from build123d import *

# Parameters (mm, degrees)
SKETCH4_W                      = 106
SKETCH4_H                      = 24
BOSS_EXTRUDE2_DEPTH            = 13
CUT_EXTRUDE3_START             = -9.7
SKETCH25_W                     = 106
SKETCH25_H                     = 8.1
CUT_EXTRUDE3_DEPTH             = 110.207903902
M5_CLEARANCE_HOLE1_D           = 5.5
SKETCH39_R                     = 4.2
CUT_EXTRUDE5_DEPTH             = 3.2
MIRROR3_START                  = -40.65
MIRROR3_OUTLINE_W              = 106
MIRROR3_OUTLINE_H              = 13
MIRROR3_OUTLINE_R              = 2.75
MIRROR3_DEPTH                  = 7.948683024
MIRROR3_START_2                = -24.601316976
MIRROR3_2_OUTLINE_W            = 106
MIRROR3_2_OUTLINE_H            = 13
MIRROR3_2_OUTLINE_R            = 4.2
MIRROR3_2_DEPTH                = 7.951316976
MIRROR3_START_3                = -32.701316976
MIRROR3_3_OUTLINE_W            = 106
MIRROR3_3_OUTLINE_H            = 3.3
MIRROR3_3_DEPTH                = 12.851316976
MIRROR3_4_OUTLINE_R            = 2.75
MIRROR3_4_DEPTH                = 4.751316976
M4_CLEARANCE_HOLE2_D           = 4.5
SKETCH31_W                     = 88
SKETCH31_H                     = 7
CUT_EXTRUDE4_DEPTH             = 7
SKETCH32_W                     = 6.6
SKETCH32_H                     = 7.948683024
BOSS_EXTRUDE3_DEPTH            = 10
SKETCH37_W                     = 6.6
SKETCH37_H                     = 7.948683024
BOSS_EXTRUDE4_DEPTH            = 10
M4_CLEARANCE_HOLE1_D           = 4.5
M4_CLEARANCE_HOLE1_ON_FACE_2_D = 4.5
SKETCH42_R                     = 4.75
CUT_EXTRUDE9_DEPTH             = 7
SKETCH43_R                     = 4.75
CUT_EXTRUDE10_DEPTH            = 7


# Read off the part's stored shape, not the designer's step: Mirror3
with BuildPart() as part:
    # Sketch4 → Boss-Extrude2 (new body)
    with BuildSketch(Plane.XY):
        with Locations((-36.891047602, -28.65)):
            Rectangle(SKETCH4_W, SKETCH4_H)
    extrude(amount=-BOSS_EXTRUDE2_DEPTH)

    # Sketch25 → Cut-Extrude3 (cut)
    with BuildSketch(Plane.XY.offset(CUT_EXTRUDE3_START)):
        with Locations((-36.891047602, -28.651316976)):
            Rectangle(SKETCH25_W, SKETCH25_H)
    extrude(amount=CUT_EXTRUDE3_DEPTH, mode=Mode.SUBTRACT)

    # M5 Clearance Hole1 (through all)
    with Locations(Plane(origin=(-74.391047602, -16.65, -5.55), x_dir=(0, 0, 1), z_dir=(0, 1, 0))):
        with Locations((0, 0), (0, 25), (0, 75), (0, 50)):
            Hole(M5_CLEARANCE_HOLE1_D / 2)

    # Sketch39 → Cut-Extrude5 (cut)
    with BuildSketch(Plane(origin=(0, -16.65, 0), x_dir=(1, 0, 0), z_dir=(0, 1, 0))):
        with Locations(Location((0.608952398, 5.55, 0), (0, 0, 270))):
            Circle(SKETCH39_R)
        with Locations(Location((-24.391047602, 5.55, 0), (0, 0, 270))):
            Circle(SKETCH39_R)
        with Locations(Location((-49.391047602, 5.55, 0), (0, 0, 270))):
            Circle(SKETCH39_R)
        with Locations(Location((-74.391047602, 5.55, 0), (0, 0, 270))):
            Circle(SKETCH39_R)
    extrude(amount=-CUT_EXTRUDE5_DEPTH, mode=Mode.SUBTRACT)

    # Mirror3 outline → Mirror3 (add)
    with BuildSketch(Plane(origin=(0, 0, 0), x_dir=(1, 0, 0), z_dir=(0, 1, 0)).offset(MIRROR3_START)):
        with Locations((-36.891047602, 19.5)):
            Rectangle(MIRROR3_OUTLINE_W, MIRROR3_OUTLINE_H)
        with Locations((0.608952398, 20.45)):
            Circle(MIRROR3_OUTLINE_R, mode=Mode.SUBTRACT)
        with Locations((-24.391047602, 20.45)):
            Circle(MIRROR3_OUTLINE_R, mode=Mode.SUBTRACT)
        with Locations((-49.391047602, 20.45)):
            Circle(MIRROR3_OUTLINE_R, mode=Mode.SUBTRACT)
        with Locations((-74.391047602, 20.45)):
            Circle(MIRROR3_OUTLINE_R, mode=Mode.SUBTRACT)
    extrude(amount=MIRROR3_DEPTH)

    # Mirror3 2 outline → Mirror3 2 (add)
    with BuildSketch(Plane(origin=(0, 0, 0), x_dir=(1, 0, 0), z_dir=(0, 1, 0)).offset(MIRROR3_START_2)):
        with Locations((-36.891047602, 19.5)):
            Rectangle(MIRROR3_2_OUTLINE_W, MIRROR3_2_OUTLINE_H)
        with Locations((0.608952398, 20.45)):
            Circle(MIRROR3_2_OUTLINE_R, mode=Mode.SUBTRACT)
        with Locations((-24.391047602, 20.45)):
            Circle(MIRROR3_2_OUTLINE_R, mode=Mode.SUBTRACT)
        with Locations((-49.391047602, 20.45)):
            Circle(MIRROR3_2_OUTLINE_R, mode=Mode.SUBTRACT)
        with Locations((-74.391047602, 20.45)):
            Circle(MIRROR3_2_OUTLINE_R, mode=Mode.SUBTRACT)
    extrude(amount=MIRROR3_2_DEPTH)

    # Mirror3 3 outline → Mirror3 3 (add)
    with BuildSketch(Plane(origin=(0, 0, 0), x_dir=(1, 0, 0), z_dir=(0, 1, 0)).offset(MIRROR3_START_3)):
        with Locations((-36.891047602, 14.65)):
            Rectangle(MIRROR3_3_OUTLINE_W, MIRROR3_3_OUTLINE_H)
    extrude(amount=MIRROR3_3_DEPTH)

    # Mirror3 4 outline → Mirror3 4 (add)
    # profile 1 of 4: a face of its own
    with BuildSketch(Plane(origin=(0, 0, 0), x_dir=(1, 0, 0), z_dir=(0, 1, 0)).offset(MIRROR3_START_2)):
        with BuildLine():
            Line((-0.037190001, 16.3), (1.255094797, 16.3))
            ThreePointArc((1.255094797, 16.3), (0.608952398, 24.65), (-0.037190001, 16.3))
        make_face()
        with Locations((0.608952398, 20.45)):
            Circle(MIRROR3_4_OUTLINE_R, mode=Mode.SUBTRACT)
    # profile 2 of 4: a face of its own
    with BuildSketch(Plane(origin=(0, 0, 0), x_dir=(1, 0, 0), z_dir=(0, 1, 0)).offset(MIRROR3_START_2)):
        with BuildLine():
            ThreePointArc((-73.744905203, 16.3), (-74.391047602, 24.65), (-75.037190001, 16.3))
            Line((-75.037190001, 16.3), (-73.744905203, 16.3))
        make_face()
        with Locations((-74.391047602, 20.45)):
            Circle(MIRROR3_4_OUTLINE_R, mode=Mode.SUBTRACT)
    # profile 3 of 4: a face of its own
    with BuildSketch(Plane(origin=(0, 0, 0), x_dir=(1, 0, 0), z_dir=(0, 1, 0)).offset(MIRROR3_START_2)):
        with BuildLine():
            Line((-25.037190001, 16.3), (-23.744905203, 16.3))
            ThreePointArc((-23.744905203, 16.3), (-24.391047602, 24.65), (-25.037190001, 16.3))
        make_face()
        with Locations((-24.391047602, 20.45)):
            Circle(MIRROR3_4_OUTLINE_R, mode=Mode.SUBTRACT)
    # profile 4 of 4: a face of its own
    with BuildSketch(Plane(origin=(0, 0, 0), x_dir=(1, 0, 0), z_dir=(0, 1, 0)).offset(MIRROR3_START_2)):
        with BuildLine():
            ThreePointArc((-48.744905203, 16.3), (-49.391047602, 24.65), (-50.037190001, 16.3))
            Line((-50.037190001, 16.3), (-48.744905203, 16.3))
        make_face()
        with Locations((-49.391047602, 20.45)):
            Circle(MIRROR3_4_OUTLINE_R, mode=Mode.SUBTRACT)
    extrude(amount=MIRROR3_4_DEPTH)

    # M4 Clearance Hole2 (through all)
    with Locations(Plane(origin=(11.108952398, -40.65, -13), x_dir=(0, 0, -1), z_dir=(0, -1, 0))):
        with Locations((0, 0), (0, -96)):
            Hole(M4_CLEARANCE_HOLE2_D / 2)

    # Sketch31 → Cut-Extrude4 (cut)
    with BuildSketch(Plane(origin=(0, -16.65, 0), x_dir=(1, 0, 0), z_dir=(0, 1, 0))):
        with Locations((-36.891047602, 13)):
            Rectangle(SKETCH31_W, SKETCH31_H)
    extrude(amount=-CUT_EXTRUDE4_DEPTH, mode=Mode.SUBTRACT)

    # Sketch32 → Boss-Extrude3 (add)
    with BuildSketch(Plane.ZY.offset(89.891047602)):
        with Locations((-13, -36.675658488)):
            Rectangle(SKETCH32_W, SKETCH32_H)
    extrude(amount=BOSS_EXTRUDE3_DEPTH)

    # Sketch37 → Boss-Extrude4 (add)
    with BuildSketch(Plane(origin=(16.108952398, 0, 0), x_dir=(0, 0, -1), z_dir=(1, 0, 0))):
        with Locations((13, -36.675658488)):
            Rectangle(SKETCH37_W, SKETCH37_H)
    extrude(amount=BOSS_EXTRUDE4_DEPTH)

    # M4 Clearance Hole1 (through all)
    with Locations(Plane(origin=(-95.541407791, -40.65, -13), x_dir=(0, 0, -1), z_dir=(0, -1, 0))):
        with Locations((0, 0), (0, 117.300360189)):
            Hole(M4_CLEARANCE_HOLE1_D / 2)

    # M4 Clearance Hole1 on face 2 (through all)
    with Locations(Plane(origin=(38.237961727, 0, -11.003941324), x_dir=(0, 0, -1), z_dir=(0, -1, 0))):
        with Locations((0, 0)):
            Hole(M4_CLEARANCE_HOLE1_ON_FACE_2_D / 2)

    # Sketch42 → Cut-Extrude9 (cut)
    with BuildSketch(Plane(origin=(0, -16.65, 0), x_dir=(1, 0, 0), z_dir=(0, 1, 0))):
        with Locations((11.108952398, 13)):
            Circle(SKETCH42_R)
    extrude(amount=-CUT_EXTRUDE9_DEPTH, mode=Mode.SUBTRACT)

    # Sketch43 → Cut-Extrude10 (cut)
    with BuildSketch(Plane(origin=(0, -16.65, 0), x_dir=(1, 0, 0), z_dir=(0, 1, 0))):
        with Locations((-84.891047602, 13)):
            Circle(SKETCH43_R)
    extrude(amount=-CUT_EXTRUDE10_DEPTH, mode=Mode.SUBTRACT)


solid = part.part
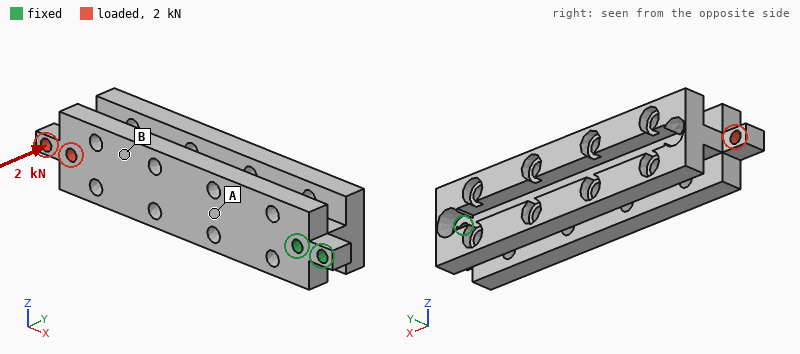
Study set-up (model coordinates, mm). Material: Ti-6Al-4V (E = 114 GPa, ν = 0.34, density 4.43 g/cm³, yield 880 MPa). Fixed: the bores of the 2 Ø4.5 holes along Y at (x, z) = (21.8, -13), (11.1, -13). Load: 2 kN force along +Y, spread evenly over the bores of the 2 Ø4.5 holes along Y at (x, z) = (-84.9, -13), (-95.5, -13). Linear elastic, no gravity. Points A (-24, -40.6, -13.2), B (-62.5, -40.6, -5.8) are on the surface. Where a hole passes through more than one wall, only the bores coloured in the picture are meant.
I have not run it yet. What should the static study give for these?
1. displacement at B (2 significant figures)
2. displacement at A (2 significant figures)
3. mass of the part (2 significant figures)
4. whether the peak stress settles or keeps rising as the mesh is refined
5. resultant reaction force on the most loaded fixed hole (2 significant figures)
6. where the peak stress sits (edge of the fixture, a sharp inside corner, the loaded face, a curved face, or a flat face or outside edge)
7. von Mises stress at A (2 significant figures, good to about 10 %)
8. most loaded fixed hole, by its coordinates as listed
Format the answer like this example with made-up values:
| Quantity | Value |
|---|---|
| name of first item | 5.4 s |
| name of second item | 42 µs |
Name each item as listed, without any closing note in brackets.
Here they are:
| Quantity | Value |
|---|---|
| displacement at B | 0.42 mm |
| displacement at A | 0.15 mm |
| mass of the part | 180 g |
| whether the peak stress settles or keeps rising as the mesh is refined | keeps rising |
| resultant reaction force on the most loaded fixed hole | 2.7 kN |
| where the peak stress sits | edge of the fixture |
| von Mises stress at A | 80 MPa |
| most loaded fixed hole, by its coordinates as listed | (11.1, -13) |
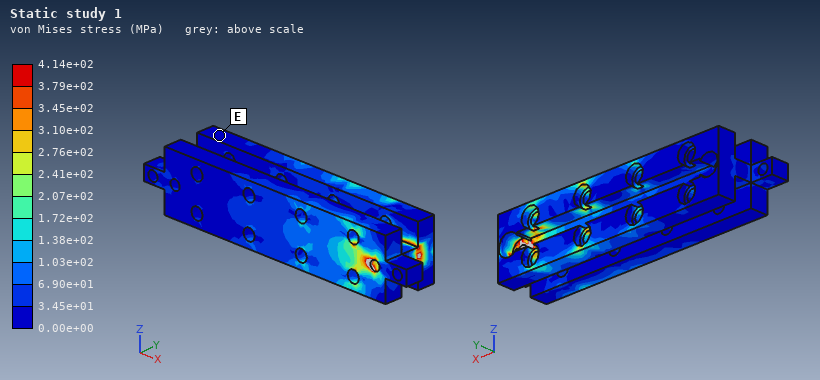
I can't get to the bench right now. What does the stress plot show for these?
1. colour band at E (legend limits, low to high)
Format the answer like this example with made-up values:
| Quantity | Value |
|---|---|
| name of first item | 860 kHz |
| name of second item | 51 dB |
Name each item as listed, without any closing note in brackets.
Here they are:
| Quantity | Value |
|---|---|
| colour band at E | 0.00e+00 to 3.45e+01 MPa |
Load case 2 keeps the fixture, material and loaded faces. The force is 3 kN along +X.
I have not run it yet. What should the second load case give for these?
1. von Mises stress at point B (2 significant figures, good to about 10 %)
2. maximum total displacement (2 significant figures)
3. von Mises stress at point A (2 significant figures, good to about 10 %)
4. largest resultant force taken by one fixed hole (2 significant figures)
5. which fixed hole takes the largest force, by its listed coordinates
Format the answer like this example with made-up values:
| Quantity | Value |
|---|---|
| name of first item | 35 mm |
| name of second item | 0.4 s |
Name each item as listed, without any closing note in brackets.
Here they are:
| Quantity | Value |
|---|---|
| von Mises stress at point B | 11 MPa |
| maximum total displacement | 32 µm |
| von Mises stress at point A | 13 MPa |
| largest resultant force taken by one fixed hole | 2.8 kN |
| which fixed hole takes the largest force, by its listed coordinates | (11.1, -13) |
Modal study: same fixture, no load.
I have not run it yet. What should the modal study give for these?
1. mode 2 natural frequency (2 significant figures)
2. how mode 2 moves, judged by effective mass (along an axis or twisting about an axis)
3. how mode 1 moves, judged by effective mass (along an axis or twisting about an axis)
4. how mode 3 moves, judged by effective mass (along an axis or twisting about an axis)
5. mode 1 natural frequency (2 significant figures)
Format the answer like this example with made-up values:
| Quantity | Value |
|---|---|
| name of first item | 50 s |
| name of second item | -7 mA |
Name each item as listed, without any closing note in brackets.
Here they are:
| Quantity | Value |
|---|---|
| mode 2 natural frequency | 1300 Hz |
| how mode 2 moves, judged by effective mass | along Y |
| how mode 1 moves, judged by effective mass | along Z |
| how mode 3 moves, judged by effective mass | twisting about X |
| mode 1 natural frequency | 1000 Hz |
